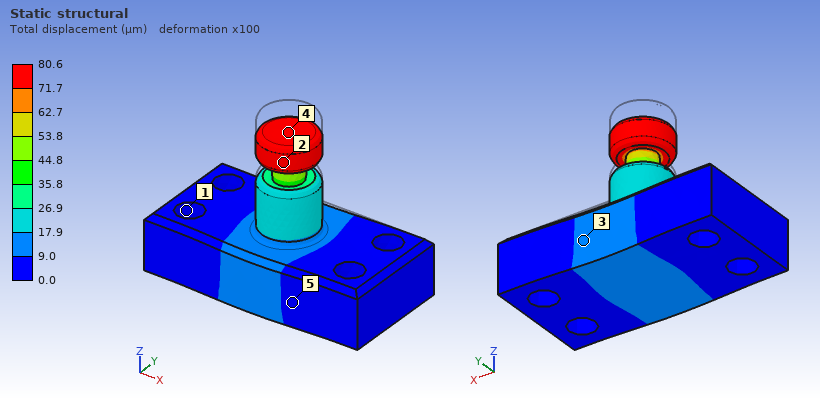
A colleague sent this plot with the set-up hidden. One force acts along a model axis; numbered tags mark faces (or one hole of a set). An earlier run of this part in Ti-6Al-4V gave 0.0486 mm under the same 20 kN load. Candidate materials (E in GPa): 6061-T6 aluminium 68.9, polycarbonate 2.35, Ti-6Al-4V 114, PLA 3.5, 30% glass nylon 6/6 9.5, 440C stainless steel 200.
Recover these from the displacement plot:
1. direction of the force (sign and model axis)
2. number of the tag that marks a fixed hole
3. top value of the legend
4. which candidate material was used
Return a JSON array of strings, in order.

["-Z", "1", "80.6 µm", "6061-T6 aluminium"]
